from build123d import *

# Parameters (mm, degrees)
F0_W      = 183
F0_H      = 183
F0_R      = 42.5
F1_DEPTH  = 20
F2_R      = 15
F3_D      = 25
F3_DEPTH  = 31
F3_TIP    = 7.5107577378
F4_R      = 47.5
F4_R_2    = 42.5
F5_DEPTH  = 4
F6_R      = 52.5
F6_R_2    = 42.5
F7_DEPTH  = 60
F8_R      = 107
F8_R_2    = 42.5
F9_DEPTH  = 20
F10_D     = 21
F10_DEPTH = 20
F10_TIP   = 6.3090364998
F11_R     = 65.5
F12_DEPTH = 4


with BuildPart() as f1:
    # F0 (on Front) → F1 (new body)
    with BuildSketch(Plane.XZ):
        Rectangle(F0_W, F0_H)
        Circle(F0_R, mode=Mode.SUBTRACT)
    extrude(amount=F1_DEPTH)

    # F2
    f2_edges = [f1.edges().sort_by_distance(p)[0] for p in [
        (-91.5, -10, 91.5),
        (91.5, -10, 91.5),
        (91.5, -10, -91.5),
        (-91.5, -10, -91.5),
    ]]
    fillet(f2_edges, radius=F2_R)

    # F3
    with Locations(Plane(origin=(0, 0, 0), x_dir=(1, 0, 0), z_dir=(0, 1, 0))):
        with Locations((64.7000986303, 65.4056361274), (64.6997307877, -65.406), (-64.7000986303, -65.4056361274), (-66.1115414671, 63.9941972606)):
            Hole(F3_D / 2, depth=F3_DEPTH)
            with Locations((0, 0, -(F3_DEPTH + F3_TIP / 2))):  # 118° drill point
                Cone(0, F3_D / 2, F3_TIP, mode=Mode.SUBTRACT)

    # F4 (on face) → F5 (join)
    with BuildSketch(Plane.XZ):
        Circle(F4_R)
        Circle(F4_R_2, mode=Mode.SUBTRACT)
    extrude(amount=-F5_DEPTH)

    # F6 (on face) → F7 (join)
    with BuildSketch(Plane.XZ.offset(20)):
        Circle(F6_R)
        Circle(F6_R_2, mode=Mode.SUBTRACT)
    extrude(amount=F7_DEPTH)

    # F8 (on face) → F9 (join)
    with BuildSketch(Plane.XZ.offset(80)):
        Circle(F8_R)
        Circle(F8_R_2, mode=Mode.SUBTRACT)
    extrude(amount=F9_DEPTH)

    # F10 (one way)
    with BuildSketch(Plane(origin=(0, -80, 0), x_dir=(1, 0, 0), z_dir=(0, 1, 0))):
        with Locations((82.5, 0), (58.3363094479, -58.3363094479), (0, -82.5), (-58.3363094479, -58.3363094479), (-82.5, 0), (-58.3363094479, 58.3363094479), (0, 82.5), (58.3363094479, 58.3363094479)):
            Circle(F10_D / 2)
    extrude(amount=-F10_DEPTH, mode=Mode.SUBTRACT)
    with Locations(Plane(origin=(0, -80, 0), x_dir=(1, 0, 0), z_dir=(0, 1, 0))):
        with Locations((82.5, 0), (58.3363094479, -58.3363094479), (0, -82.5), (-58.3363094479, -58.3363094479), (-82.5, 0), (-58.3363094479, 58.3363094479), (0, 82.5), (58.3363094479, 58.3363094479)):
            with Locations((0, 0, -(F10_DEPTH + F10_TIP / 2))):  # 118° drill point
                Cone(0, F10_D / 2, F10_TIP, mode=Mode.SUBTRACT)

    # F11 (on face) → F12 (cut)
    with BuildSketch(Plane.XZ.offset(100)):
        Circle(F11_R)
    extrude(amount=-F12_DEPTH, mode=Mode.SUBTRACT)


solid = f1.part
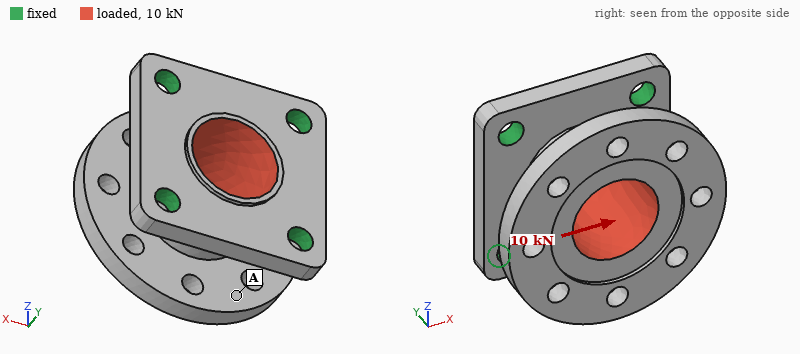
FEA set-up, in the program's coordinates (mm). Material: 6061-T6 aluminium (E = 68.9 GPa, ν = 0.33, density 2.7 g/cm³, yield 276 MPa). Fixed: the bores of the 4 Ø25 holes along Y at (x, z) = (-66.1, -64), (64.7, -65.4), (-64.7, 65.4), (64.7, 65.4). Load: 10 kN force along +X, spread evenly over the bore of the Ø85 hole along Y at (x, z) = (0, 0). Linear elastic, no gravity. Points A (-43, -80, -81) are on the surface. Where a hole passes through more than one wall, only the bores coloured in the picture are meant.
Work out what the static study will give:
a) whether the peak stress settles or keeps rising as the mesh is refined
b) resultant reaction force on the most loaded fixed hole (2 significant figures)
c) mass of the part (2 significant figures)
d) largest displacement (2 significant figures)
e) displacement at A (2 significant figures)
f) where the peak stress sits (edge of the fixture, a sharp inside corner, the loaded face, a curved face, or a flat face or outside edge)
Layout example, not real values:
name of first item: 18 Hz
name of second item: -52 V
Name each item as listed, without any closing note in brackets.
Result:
whether the peak stress settles or keeps rising as the mesh is refined: keeps rising
resultant reaction force on the most loaded fixed hole: 3.1 kN
mass of the part: 3.3 kg
largest displacement: 29 µm
displacement at A: 20 µm
where the peak stress sits: edge of the fixture
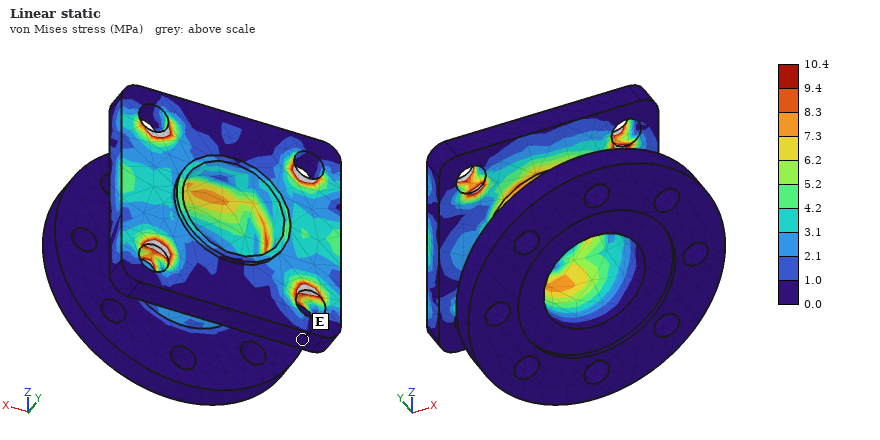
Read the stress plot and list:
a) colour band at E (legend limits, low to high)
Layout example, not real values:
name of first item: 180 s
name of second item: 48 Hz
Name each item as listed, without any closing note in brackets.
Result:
colour band at E: 0.0 to 1.0 MPa
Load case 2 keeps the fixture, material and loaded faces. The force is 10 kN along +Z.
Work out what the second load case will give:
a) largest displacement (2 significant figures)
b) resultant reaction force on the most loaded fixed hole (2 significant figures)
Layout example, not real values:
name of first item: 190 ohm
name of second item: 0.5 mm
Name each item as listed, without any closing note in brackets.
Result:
largest displacement: 28 µm
resultant reaction force on the most loaded fixed hole: 3.1 kN
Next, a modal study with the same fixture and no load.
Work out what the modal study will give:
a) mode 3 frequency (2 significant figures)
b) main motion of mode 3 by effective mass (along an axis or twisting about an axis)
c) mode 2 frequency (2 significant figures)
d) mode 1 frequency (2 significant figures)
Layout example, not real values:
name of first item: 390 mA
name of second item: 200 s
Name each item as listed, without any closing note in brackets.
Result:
mode 3 frequency: 2000 Hz
main motion of mode 3 by effective mass: along Y
mode 2 frequency: 1400 Hz
mode 1 frequency: 1400 Hz
